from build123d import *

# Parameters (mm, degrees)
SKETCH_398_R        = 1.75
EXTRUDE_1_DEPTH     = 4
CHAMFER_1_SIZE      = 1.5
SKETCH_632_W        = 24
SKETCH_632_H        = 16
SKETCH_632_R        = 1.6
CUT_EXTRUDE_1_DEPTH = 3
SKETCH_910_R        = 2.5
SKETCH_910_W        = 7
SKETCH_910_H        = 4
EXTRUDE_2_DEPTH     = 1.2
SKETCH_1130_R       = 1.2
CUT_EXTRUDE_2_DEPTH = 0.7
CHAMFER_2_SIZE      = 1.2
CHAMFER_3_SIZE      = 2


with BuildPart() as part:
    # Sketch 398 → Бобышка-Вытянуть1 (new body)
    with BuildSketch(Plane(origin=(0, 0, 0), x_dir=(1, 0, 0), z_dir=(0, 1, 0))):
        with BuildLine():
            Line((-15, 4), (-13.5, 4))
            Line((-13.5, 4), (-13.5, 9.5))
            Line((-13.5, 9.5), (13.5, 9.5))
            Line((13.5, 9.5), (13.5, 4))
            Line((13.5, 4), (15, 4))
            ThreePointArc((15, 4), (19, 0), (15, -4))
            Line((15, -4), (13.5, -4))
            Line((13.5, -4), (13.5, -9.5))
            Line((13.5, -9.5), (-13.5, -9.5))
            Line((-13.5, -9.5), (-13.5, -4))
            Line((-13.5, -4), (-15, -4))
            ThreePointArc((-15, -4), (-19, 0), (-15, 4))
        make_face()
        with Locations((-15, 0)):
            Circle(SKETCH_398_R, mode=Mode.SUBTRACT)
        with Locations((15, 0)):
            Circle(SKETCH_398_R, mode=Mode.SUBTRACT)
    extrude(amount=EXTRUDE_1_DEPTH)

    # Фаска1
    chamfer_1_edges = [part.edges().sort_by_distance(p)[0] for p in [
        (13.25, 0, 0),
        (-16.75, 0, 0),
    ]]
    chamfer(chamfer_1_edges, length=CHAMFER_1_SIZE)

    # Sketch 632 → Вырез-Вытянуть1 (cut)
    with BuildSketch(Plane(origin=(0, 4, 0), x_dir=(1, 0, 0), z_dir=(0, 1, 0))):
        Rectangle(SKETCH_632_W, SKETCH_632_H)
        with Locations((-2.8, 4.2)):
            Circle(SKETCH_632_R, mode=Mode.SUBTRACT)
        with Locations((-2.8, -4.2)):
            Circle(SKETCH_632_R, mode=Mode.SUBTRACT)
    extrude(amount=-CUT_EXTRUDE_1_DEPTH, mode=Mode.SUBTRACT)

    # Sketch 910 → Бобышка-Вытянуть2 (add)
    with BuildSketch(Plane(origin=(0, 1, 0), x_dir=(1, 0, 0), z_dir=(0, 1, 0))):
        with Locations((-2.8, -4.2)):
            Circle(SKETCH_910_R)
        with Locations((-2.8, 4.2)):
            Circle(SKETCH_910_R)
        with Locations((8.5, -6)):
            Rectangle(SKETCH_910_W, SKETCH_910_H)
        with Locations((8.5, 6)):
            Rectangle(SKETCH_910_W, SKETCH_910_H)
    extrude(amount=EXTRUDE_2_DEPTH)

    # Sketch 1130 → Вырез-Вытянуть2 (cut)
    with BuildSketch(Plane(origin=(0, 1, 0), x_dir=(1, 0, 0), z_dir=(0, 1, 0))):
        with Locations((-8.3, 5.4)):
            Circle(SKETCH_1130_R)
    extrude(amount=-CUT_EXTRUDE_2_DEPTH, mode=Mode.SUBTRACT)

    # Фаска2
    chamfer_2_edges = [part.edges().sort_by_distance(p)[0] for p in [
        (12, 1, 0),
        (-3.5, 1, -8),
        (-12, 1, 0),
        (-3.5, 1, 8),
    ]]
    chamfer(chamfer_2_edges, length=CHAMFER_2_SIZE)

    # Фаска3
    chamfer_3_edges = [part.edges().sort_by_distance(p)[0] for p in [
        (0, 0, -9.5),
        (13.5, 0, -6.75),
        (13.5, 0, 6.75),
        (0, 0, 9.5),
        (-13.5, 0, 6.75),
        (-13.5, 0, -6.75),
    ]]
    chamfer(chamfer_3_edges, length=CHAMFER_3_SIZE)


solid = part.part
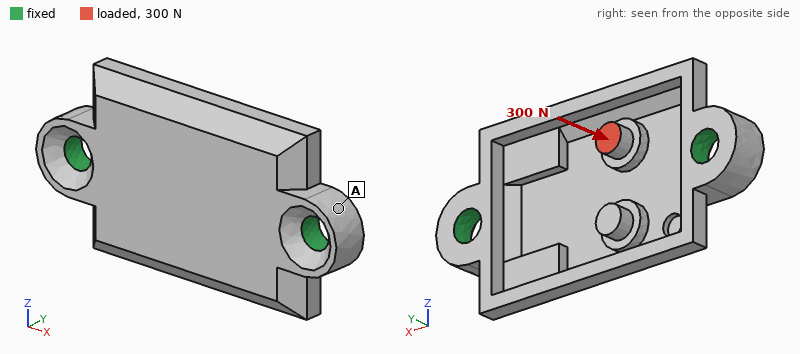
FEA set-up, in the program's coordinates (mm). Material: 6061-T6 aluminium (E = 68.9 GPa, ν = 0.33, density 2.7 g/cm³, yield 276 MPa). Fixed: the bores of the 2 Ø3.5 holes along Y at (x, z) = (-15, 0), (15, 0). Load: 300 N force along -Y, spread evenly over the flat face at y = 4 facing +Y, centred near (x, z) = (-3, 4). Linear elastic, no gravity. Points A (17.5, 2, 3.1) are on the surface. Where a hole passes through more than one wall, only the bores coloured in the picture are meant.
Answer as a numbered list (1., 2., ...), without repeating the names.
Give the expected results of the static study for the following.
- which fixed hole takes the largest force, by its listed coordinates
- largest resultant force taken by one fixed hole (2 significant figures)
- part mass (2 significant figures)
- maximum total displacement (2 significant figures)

1. (-15, 0)
2. 220 N
3. 3.0 g
4. 83 µm
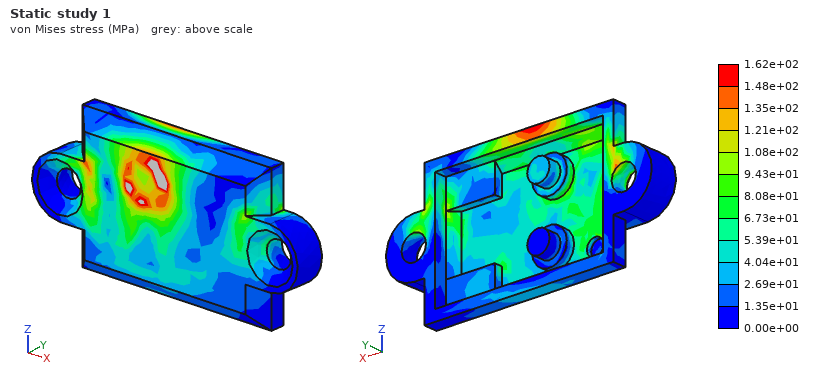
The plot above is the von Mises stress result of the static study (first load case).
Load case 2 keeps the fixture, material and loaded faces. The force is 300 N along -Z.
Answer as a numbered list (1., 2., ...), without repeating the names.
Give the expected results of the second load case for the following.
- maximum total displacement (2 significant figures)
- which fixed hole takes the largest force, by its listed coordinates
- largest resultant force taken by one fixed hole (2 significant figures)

1. 73 µm
2. (-15, 0)
3. 190 N
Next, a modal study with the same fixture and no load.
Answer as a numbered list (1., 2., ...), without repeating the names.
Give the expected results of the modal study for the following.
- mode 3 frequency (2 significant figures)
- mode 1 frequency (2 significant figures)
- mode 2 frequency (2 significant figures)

1. 20 kHz
2. 12 kHz
3. 12 kHz
